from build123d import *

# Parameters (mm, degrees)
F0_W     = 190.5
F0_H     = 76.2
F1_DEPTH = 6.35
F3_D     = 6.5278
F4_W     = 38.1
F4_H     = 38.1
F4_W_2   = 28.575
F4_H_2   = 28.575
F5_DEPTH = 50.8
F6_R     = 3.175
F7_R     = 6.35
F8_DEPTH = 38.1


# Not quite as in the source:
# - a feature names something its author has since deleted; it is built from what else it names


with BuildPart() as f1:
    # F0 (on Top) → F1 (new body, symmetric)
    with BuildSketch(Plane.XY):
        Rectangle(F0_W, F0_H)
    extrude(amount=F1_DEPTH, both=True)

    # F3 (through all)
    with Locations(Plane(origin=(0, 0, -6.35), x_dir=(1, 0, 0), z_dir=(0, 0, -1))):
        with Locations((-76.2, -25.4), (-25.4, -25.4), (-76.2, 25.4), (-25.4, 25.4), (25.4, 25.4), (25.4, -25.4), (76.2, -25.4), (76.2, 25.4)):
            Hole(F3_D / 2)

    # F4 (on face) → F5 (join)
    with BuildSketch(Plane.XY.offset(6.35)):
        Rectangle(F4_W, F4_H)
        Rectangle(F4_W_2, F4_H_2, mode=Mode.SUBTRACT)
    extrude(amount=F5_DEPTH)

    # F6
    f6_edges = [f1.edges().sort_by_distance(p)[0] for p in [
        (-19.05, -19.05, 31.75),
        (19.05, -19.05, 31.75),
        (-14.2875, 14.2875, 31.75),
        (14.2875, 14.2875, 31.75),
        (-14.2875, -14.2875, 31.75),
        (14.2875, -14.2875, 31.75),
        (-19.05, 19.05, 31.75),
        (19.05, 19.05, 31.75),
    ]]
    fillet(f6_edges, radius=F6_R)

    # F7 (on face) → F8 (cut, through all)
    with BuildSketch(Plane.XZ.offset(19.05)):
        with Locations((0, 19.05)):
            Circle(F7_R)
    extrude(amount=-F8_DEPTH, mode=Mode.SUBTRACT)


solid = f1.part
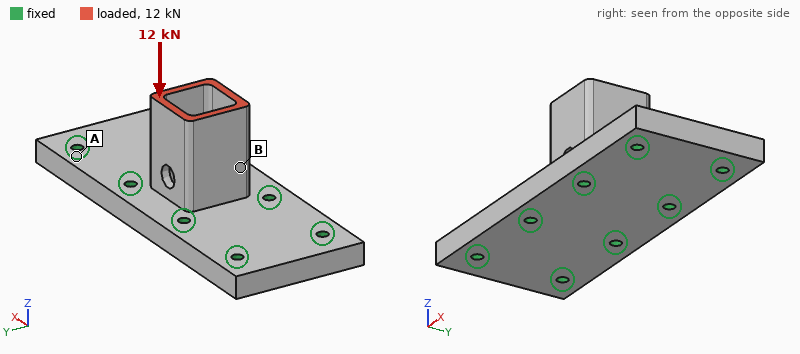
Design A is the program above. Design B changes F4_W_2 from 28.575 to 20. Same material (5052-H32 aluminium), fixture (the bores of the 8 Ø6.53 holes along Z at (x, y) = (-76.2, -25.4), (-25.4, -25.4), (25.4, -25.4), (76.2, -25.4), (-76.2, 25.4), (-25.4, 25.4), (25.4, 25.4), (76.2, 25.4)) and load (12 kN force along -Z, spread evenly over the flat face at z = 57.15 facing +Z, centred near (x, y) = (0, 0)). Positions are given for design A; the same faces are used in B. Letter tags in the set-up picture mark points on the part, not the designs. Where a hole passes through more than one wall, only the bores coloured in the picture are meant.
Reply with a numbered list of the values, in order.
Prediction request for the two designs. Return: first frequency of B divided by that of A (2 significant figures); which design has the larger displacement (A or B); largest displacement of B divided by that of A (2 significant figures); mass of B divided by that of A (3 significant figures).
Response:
1. 0.92
2. A
3. 0.82
4. 1.06
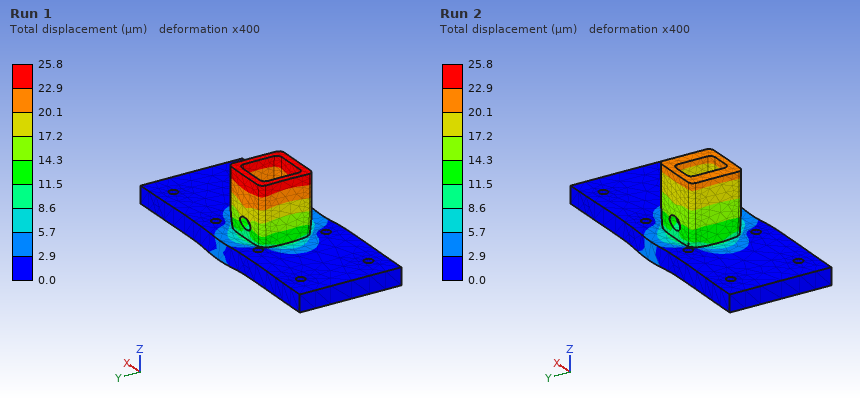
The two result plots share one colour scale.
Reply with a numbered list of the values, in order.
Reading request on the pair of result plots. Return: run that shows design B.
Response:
1. Run 2
